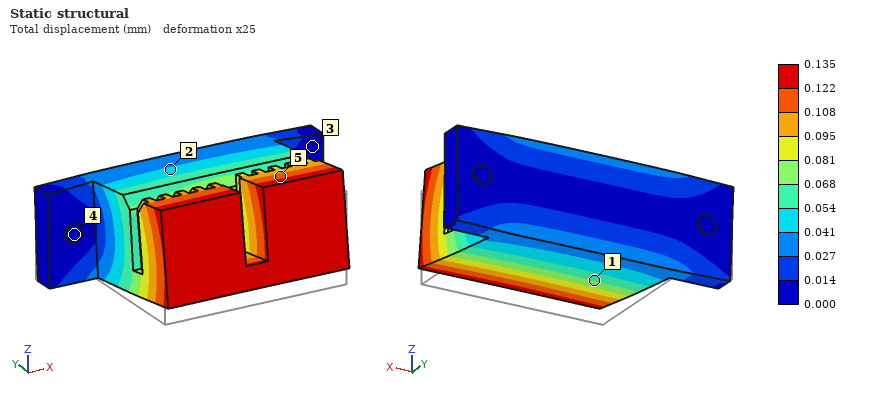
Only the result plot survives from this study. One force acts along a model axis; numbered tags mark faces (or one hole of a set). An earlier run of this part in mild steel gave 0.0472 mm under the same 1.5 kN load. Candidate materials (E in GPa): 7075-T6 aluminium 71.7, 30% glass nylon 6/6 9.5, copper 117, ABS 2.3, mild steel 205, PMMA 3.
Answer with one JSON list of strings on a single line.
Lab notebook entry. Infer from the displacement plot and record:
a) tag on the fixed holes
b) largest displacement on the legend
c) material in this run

["4", "0.135 mm", "7075-T6 aluminium"]
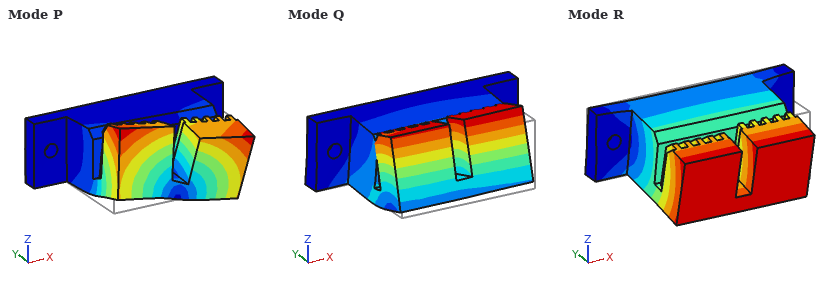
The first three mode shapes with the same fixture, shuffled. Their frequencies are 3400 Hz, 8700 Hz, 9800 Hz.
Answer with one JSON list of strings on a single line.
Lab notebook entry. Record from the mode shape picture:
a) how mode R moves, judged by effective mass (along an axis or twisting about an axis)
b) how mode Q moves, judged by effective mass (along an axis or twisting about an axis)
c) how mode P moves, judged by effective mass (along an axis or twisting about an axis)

["along Z", "along Y", "along X"]
